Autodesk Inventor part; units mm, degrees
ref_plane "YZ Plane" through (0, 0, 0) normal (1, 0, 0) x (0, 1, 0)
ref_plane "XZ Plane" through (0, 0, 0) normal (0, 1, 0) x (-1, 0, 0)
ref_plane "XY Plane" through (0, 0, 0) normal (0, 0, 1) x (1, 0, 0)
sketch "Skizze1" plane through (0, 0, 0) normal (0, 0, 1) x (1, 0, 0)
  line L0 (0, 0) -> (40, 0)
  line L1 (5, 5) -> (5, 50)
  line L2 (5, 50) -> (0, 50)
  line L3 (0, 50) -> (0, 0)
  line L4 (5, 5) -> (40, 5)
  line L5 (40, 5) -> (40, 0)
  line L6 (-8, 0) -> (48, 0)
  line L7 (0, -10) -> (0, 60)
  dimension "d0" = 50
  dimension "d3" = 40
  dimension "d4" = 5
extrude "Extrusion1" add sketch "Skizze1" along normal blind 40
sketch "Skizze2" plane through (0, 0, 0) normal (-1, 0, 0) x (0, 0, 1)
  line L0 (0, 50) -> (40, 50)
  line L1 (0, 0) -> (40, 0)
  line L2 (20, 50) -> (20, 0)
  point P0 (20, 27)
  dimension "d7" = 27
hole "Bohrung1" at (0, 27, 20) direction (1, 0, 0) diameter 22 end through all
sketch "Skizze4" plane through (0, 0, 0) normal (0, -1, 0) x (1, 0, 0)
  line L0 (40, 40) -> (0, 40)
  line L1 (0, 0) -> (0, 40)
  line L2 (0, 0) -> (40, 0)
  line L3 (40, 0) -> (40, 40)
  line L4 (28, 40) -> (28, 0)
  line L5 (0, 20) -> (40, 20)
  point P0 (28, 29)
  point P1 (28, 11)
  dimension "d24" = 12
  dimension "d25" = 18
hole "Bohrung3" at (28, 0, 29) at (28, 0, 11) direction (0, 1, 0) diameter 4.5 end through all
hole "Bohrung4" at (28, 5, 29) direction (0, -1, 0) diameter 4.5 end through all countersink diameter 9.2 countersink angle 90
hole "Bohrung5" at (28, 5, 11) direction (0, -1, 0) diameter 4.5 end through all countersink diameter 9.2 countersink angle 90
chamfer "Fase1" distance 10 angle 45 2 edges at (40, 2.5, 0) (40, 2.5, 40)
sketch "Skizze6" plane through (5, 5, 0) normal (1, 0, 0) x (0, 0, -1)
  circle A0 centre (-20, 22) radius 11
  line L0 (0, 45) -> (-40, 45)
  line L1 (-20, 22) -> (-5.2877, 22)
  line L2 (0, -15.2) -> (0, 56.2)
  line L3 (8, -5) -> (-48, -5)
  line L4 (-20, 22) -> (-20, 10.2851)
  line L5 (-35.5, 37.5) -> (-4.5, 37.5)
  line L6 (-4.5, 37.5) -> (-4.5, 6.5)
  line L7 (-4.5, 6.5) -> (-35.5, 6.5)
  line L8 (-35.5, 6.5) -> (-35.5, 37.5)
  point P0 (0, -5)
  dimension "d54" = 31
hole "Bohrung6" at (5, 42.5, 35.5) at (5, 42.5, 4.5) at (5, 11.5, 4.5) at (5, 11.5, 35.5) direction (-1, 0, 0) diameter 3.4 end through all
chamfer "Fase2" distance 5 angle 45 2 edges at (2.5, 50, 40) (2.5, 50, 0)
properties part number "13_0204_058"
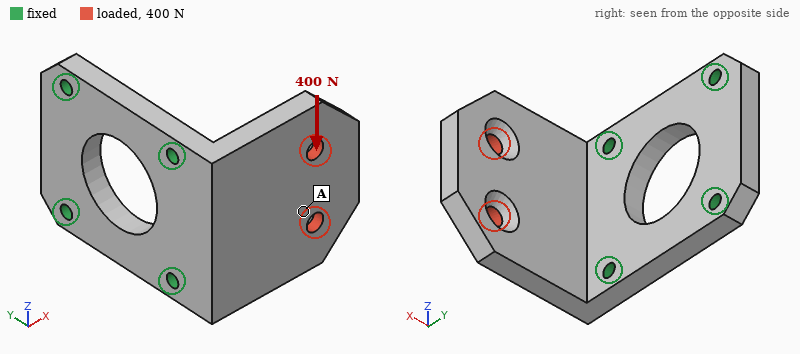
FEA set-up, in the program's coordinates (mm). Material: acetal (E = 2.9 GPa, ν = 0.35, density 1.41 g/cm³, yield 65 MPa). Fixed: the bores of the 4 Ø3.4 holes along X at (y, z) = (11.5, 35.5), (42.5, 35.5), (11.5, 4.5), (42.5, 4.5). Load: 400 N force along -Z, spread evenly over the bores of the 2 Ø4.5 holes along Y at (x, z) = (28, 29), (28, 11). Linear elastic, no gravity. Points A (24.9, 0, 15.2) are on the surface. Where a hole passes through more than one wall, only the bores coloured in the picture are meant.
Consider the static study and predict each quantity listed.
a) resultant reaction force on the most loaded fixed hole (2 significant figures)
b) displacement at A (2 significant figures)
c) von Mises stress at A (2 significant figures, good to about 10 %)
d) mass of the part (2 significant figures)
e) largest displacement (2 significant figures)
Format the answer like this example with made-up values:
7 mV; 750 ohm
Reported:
400 N; 0.26 mm; 5.3 MPa; 20 g; 0.46 mm
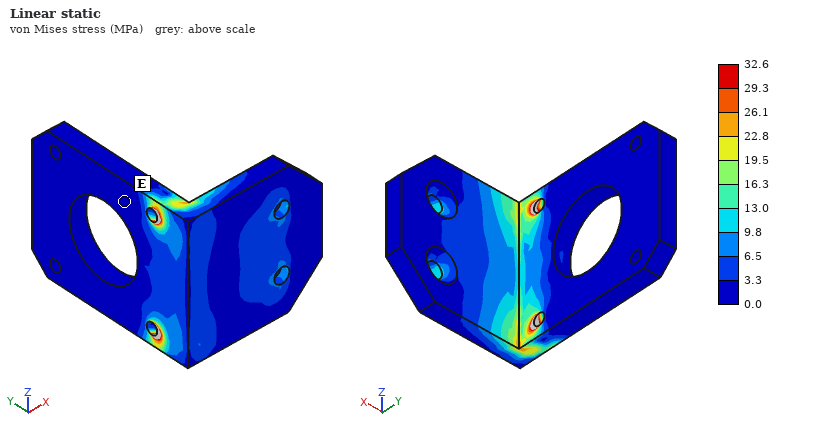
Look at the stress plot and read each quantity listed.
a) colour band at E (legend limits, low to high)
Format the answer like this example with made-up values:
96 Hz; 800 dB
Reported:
0.0 to 3.3 MPa
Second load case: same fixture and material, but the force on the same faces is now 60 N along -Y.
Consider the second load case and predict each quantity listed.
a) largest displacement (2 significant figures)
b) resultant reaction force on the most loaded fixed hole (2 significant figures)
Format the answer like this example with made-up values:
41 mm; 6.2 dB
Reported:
0.88 mm; 31 N
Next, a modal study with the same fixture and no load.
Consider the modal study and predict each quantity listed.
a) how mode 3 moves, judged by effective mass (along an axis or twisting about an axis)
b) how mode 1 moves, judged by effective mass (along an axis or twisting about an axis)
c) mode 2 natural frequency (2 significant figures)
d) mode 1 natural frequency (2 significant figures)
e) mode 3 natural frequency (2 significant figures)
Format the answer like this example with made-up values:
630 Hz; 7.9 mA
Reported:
along Z; along Y; 1800 Hz; 670 Hz; 2500 Hz
